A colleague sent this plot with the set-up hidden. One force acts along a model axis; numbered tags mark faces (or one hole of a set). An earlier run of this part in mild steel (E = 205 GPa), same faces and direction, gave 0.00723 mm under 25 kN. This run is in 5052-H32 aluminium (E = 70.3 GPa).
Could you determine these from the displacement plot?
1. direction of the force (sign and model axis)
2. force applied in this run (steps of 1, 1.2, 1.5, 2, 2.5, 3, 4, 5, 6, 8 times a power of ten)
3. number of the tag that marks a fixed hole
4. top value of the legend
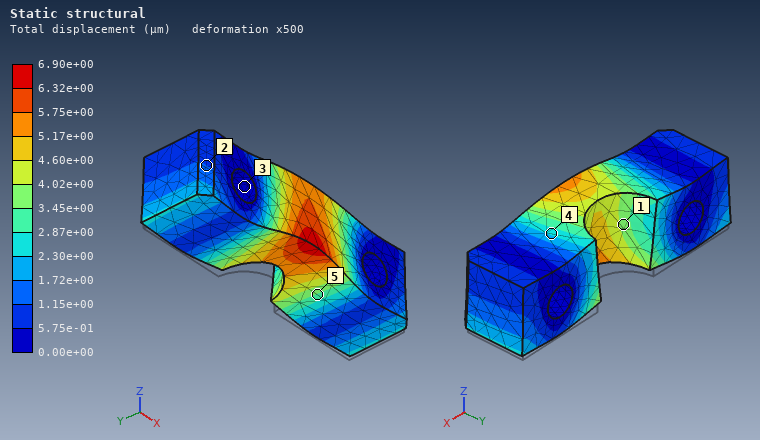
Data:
+Z
8 kN
3
6.90e+00 µm
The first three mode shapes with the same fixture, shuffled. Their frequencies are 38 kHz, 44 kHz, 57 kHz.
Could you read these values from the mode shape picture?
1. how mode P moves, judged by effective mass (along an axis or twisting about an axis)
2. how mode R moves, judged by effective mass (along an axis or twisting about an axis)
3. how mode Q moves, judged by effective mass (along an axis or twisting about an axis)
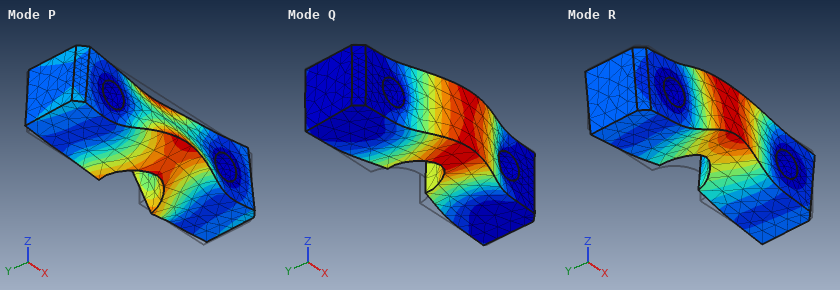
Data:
twisting about X
along Z
along Y
